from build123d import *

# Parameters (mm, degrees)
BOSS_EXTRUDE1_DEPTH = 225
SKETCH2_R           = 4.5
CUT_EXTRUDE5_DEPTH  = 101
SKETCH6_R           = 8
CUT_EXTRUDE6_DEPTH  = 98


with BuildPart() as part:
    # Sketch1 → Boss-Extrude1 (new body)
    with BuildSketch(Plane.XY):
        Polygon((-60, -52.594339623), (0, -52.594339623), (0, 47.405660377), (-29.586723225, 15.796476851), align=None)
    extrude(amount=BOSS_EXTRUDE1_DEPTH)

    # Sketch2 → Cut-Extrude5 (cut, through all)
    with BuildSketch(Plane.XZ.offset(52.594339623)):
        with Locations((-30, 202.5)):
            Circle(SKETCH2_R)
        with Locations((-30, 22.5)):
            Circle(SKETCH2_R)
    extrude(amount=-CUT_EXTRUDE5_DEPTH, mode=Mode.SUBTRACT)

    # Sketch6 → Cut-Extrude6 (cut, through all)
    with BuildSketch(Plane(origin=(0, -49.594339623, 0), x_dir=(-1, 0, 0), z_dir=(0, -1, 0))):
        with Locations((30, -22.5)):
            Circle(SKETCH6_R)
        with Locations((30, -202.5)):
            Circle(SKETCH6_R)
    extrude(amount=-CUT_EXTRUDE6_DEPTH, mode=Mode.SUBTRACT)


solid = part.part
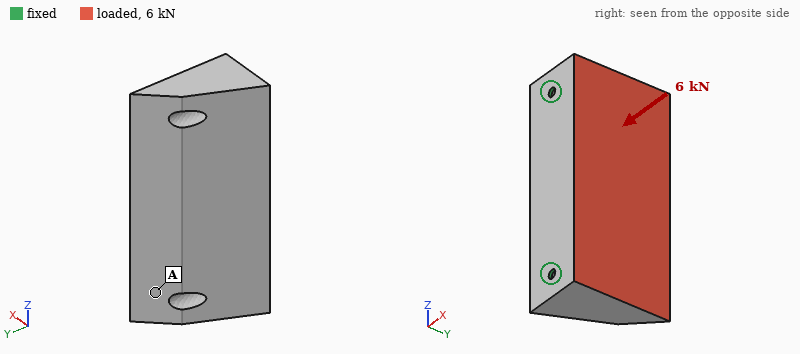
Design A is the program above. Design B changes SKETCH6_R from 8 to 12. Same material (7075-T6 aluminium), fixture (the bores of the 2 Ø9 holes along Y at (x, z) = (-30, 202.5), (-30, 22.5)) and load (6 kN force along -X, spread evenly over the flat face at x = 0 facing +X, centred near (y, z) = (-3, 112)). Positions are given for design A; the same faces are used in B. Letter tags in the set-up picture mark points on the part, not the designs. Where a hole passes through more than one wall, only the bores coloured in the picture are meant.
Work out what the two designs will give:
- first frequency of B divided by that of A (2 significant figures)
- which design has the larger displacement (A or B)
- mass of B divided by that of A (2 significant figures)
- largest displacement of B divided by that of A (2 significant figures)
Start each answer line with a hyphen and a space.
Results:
- 0.80
- B
- 0.96
- 1.6
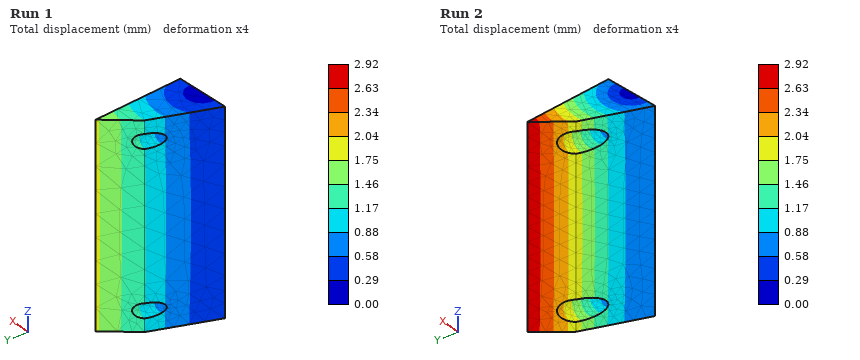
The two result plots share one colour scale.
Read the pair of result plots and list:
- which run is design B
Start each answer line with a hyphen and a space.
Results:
- Run 2
